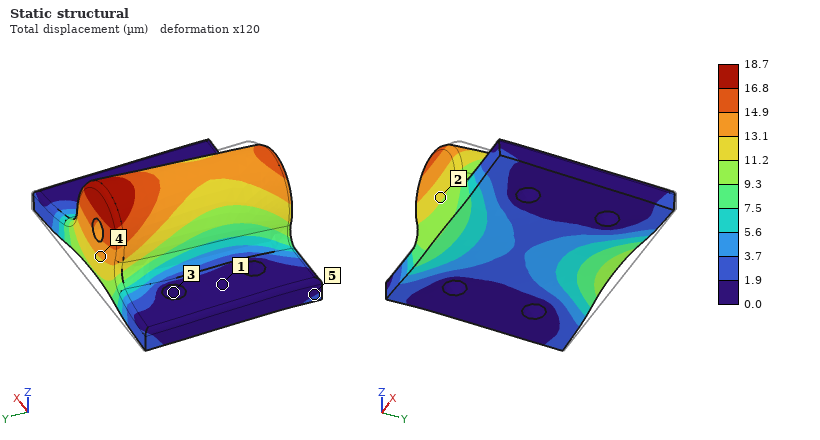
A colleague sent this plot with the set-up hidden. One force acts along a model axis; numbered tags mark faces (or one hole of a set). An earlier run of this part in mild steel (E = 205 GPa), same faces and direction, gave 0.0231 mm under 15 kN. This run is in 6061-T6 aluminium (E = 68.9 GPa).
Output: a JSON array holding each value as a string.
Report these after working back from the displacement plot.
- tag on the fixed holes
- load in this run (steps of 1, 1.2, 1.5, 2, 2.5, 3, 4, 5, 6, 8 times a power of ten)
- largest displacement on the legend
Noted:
["3", "4 kN", "18.7 µm"]
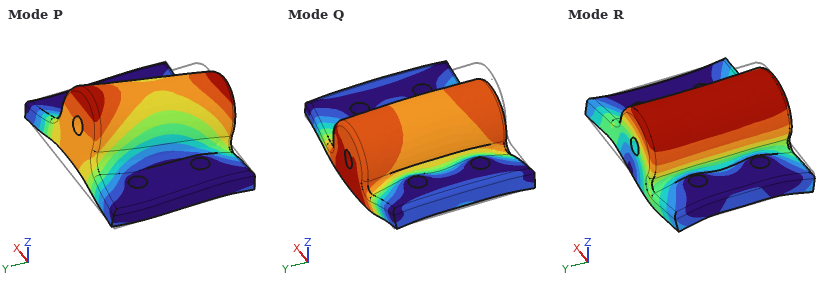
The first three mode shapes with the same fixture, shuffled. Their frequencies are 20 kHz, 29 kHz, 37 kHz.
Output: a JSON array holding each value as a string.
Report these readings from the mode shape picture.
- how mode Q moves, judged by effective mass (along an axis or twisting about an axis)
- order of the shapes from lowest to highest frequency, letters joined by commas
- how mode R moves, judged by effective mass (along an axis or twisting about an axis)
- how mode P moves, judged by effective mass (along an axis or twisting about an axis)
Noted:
["along Z", "P, Q, R", "along X", "along Y"]
